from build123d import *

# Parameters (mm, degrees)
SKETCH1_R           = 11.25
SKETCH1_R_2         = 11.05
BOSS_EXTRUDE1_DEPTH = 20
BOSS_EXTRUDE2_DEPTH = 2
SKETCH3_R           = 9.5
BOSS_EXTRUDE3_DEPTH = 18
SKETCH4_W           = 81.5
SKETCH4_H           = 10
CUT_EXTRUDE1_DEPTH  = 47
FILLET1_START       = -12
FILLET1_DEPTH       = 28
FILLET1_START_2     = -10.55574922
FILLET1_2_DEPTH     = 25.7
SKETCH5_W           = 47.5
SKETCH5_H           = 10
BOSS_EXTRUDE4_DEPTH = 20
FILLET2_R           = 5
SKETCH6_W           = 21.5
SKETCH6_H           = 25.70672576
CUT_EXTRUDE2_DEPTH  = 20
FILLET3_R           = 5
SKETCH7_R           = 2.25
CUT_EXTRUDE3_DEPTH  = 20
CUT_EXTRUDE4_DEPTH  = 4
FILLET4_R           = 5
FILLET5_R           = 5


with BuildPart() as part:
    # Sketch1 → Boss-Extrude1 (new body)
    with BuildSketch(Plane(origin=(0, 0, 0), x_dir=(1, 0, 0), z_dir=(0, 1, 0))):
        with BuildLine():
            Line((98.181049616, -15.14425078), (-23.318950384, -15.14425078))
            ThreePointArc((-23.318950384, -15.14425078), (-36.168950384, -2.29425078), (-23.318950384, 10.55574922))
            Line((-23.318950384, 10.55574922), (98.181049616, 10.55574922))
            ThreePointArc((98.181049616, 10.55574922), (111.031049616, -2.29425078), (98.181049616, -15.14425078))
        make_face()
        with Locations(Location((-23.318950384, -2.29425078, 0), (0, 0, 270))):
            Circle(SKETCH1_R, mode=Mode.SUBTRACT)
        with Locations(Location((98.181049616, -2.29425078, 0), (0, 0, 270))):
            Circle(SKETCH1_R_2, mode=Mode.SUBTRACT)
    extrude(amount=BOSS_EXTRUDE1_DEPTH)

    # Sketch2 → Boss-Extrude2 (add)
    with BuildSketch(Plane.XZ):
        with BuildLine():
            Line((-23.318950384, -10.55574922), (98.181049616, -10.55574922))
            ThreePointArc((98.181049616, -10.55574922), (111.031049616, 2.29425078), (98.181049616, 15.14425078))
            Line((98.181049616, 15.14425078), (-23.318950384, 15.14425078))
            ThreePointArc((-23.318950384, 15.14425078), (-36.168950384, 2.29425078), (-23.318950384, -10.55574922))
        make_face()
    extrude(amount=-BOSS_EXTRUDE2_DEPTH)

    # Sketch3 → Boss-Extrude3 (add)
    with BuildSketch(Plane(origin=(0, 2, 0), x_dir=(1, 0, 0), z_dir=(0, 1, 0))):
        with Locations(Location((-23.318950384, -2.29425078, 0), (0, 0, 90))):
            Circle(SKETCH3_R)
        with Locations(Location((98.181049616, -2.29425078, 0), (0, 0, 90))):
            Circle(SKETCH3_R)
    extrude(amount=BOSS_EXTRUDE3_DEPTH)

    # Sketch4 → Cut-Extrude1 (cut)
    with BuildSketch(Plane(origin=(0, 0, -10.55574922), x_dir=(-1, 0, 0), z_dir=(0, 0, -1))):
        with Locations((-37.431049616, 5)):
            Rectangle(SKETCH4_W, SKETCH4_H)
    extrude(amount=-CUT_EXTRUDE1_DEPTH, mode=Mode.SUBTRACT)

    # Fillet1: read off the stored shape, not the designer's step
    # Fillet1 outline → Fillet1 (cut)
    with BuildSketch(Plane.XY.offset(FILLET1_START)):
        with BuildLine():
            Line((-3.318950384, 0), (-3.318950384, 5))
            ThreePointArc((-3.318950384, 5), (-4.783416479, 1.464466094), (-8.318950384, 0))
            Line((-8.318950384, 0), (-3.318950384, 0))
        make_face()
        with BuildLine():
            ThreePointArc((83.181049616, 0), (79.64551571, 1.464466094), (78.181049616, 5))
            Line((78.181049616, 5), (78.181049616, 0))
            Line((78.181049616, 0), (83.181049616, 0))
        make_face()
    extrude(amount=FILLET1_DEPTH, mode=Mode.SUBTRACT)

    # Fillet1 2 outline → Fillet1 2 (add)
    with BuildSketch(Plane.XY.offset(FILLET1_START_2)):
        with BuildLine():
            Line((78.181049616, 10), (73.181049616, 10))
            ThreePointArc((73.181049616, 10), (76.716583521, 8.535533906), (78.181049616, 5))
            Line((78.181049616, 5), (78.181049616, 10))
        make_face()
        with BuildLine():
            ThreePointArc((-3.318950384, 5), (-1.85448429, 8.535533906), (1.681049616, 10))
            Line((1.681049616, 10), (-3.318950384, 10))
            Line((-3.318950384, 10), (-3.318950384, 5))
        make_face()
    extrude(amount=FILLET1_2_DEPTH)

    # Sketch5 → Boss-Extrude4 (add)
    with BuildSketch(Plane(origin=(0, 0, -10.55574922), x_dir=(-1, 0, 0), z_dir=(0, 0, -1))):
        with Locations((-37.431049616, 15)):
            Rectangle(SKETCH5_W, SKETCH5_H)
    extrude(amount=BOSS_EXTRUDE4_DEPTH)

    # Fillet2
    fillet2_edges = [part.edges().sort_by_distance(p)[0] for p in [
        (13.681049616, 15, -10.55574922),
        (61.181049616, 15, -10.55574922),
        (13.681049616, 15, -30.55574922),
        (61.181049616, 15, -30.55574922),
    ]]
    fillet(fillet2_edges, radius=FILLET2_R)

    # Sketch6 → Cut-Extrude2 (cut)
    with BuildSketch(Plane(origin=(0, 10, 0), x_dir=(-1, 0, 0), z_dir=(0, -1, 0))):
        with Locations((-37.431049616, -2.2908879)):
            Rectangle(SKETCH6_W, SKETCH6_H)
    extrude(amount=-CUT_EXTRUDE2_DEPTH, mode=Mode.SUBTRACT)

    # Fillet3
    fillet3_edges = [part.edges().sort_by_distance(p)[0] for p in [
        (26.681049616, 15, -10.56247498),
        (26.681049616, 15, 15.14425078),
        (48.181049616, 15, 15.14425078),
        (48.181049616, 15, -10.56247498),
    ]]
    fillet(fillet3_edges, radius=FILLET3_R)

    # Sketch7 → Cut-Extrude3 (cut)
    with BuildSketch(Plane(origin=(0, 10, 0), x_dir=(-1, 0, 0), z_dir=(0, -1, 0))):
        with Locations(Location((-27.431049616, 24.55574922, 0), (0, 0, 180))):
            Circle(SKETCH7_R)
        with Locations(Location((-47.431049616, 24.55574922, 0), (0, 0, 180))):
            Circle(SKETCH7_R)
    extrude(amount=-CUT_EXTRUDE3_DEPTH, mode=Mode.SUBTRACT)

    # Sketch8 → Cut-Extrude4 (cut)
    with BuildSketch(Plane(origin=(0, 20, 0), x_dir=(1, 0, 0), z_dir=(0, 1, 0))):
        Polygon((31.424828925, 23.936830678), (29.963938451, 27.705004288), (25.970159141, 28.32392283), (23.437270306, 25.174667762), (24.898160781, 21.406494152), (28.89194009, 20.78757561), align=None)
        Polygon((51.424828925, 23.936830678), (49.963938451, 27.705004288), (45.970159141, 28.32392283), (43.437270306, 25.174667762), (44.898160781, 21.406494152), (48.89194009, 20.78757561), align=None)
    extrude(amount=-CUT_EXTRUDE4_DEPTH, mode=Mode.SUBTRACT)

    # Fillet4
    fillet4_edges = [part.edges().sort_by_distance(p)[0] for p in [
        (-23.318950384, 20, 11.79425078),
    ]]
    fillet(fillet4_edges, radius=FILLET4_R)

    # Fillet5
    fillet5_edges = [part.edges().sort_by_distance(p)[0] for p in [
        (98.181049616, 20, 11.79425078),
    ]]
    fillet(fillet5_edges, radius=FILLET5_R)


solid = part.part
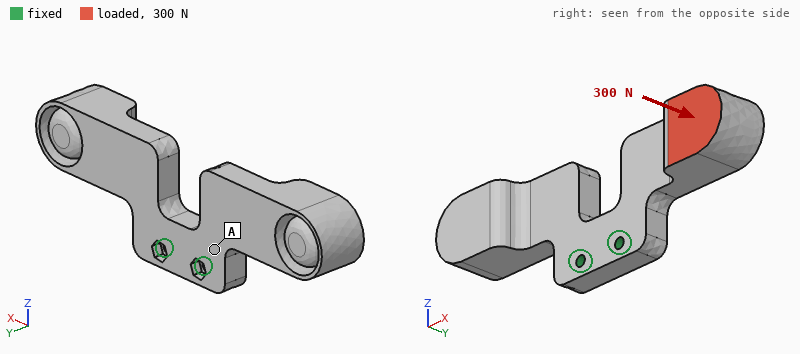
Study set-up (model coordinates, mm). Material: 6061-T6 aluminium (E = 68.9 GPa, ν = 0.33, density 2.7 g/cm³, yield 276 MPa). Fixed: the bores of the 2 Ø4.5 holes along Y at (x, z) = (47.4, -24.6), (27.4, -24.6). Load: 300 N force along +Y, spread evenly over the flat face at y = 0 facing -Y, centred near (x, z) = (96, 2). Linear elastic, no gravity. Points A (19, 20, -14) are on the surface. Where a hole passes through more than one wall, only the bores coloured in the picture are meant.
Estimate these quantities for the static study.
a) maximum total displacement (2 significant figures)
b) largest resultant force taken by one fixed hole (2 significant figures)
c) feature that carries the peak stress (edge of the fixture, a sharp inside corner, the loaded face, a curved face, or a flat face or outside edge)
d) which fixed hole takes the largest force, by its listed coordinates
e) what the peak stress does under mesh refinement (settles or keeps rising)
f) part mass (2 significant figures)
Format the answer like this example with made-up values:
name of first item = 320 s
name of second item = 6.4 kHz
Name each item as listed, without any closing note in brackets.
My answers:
maximum total displacement = 0.30 mm
largest resultant force taken by one fixed hole = 810 N
feature that carries the peak stress = edge of the fixture
which fixed hole takes the largest force, by its listed coordinates = (47.4, -24.6)
what the peak stress does under mesh refinement = keeps rising
part mass = 140 g
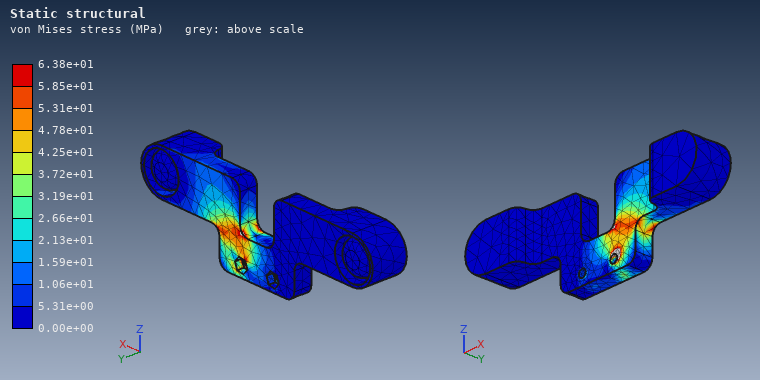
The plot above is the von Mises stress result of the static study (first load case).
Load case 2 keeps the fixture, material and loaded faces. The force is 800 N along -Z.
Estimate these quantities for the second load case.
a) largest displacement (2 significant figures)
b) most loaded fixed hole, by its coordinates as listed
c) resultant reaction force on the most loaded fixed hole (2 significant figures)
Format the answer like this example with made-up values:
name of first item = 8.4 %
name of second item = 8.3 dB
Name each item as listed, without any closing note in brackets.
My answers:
largest displacement = 0.30 mm
most loaded fixed hole, by its coordinates as listed = (47.4, -24.6)
resultant reaction force on the most loaded fixed hole = 2.5 kN
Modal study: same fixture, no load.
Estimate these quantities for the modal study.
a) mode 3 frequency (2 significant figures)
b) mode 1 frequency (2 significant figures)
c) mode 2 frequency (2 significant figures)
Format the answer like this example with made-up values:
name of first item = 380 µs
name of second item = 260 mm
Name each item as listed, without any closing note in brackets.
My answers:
mode 3 frequency = 1600 Hz
mode 1 frequency = 970 Hz
mode 2 frequency = 990 Hz
